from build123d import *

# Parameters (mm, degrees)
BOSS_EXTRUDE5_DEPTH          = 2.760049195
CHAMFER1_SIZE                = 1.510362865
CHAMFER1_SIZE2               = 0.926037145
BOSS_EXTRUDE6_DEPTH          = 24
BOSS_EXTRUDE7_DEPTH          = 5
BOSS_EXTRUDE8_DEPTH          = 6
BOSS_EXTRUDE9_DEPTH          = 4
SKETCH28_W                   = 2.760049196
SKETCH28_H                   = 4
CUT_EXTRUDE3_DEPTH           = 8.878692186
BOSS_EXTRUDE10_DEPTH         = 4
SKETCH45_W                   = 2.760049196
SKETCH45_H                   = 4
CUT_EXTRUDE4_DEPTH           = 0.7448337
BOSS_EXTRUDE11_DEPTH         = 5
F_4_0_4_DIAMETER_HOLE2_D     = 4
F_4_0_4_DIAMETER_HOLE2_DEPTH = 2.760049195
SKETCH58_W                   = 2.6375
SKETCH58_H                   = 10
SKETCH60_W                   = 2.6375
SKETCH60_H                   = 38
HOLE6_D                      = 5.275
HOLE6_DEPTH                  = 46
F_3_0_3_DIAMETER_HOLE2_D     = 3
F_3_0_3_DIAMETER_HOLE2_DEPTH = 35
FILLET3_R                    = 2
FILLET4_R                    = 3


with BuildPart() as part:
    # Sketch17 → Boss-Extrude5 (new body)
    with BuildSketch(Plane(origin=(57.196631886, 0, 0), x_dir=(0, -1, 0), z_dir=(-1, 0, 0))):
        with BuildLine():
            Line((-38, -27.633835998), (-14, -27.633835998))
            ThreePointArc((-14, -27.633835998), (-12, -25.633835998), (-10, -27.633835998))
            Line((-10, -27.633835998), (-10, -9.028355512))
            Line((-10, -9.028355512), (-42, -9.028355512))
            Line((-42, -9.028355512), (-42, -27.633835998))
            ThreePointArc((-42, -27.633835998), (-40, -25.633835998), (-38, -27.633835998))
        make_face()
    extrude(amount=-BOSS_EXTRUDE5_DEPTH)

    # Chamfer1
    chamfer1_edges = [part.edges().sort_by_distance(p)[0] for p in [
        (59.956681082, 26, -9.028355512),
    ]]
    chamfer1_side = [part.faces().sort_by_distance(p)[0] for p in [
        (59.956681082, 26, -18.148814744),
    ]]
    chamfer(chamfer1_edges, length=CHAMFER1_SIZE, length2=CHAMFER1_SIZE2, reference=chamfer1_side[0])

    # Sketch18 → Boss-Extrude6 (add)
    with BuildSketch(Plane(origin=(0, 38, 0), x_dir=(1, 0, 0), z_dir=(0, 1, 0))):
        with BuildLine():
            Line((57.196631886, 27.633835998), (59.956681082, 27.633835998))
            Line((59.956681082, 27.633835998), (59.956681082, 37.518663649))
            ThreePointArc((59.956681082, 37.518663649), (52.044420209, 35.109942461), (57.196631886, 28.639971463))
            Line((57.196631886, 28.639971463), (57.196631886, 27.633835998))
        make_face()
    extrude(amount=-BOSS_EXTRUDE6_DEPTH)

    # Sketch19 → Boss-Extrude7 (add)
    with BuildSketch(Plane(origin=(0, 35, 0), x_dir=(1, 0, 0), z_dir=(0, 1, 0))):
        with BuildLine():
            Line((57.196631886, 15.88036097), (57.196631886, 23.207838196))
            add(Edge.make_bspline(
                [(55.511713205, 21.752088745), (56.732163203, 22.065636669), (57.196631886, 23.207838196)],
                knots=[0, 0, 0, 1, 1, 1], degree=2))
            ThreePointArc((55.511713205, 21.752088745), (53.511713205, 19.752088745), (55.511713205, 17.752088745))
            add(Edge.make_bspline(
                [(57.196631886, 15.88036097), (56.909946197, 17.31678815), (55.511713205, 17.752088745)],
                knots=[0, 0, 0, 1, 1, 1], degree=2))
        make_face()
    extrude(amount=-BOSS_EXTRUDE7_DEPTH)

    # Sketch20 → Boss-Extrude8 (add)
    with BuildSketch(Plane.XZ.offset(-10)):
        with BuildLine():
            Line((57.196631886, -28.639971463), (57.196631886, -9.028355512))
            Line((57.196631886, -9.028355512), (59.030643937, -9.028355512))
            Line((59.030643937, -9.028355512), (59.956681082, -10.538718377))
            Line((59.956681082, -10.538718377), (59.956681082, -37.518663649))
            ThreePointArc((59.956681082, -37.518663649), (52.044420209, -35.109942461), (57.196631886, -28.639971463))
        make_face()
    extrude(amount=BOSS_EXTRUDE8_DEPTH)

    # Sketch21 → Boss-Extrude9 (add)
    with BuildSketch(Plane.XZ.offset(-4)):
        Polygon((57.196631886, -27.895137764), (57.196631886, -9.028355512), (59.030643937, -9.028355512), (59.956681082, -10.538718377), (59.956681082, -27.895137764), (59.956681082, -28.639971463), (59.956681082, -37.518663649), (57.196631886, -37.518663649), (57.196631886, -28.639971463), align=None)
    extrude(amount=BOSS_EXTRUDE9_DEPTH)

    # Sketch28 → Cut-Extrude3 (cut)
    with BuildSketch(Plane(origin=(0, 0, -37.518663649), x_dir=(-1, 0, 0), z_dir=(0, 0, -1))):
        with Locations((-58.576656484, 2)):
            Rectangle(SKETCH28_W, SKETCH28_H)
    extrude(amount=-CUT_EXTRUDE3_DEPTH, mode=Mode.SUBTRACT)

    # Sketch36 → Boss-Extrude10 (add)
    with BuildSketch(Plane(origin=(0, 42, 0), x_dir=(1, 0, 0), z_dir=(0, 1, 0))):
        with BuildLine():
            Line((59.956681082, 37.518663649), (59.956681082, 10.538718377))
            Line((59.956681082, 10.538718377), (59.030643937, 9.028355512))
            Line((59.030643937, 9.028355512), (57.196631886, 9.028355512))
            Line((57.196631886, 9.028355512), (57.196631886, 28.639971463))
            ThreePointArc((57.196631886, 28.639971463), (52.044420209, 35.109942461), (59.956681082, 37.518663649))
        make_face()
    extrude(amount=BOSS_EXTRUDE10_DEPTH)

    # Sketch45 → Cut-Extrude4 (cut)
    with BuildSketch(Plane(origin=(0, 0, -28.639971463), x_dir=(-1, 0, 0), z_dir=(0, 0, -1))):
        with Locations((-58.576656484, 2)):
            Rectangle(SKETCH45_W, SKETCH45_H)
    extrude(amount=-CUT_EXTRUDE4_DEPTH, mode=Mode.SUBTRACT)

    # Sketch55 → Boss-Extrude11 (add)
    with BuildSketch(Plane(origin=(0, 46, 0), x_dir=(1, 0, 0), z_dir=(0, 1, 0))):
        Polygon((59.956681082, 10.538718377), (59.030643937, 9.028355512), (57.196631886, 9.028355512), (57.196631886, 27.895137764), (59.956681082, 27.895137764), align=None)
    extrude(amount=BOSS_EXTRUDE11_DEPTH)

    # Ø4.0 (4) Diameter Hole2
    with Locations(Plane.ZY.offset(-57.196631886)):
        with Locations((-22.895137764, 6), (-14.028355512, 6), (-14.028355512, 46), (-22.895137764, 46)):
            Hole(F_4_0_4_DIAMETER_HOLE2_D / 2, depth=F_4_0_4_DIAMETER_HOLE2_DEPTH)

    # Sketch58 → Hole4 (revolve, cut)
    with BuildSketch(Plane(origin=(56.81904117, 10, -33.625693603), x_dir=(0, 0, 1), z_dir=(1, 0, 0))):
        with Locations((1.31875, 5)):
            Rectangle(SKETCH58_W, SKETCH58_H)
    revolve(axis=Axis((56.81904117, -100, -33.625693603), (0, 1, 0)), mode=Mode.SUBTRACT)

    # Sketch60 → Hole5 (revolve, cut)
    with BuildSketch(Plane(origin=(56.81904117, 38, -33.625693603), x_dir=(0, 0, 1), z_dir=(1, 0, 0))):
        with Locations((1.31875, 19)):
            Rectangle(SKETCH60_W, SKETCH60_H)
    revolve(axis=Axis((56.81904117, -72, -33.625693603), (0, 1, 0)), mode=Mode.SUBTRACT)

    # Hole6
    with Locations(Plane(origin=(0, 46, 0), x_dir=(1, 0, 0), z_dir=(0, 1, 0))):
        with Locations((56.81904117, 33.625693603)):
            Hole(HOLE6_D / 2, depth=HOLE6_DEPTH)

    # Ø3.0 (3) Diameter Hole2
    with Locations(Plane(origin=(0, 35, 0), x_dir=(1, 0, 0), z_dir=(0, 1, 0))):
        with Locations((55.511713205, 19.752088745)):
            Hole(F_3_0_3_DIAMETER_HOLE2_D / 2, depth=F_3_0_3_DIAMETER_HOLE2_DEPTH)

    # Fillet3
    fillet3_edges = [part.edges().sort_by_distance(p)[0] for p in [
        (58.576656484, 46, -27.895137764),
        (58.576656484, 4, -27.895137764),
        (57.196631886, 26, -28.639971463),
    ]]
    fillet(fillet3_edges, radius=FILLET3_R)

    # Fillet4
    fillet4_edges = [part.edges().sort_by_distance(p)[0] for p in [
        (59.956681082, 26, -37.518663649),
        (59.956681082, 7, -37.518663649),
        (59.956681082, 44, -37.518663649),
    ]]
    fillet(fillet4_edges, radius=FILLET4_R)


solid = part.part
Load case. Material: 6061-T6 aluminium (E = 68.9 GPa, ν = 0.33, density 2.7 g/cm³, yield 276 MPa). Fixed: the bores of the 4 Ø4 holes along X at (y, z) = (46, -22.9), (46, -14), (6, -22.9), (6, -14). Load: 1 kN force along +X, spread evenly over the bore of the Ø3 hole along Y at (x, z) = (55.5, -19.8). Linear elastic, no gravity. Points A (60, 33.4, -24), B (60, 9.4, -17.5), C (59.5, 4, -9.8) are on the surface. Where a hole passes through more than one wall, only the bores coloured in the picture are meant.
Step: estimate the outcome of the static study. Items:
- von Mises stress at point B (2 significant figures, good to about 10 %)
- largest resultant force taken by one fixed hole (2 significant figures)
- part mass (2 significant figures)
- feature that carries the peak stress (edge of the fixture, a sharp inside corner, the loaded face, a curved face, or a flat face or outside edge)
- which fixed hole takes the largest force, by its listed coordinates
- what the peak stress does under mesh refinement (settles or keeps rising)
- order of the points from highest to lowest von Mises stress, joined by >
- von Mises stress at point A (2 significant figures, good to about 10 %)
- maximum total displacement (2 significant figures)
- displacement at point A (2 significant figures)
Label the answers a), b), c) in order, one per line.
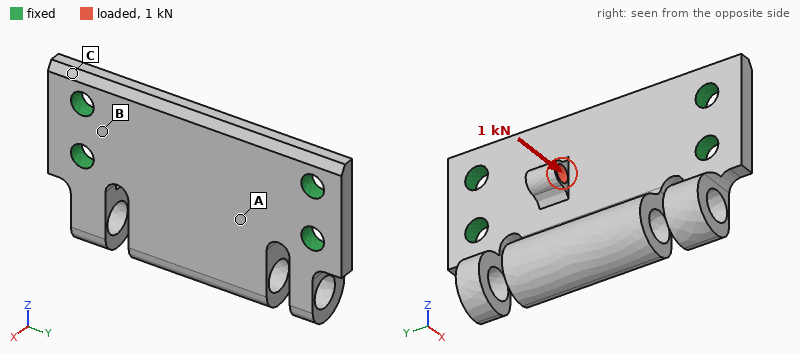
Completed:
a) 56 MPa
b) 450 N
c) 11 g
d) edge of the fixture
e) (46, -22.9)
f) keeps rising
g) A > B > C
h) 94 MPa
i) 80 µm
j) 59 µm
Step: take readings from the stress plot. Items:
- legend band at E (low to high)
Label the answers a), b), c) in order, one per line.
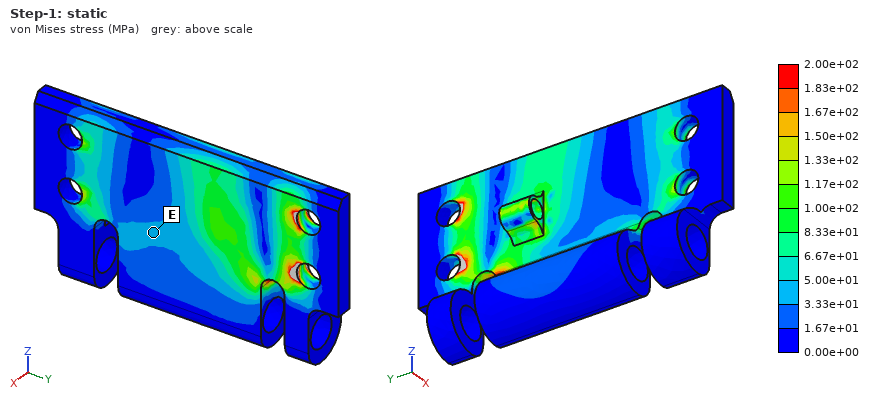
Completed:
a) 3.33e+01 to 5.00e+01 MPa
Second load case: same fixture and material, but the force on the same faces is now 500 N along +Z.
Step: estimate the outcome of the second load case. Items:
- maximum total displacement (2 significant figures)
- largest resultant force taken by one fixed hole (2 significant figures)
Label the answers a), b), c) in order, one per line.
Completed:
a) 35 µm
b) 270 N
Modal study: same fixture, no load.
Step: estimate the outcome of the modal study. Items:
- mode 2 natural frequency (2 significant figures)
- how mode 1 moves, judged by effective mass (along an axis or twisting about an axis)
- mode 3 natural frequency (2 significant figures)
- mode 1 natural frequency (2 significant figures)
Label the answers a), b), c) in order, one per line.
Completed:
a) 8400 Hz
b) along X
c) 8700 Hz
d) 4100 Hz
